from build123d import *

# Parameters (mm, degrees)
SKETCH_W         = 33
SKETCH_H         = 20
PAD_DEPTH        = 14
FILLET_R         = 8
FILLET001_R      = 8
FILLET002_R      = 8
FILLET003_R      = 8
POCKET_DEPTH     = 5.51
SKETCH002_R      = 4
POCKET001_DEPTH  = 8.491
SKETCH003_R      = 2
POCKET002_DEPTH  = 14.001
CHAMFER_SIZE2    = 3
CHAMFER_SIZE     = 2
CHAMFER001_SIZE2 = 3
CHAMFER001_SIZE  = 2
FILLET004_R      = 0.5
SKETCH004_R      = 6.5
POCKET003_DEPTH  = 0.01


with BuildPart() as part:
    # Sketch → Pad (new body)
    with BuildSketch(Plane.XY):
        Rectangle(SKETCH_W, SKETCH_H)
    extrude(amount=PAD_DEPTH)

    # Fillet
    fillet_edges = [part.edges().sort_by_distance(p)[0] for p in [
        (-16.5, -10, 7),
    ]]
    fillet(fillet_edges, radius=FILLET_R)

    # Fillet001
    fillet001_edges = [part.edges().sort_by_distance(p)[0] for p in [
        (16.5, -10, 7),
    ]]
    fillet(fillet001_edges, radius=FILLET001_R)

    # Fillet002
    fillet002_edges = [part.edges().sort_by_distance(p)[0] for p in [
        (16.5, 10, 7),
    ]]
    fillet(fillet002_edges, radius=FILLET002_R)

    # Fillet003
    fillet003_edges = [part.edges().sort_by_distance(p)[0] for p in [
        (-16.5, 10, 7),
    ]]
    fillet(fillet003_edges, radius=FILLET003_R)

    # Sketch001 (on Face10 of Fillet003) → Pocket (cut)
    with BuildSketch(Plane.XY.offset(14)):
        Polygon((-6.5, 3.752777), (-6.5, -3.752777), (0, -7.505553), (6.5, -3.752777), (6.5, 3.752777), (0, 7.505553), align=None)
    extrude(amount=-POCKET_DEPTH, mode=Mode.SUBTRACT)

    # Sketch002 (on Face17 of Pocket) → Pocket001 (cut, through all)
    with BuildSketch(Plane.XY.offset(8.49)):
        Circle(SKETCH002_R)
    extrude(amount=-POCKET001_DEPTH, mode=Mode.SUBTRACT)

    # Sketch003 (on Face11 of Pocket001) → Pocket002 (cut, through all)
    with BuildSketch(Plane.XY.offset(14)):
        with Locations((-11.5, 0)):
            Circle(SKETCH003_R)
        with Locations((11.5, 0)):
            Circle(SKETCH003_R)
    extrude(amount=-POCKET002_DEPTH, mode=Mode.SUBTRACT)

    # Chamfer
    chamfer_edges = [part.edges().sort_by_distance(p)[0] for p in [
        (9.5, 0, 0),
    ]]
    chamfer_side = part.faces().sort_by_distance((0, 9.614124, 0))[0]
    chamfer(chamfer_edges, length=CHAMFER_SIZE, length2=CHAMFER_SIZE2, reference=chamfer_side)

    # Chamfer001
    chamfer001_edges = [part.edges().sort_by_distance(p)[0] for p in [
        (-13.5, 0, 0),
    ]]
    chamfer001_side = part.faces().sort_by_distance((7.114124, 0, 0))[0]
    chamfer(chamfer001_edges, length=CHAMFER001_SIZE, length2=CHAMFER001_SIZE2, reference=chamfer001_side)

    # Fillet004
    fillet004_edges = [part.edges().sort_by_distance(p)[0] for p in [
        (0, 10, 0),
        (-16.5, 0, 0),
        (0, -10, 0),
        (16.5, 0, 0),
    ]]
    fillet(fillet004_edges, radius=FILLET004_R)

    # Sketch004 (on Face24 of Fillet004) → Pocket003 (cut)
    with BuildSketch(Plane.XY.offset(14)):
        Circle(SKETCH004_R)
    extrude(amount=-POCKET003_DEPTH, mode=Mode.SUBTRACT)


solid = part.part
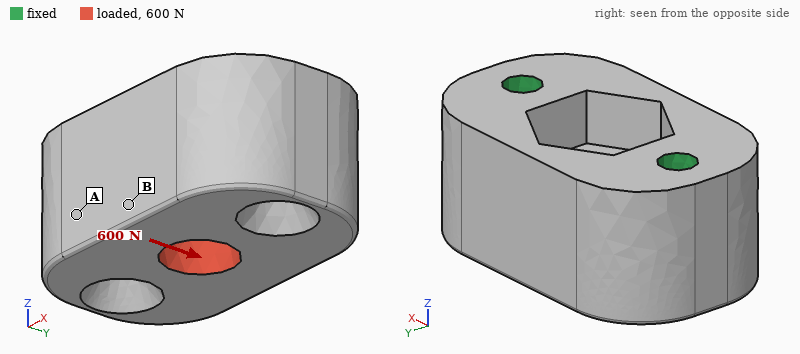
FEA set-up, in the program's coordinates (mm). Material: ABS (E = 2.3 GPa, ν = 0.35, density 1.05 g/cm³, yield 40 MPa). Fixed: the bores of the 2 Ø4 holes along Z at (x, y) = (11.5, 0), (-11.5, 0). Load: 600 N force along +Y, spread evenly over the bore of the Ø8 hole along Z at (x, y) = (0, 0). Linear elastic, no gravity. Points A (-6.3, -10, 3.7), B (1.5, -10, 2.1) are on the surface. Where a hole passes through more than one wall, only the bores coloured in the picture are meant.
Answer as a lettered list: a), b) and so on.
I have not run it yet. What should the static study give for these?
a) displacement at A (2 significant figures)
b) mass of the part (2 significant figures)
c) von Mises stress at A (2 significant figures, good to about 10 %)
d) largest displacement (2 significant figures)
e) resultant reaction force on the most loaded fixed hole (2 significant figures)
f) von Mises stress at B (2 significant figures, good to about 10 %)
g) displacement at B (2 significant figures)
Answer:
a) 23 µm
b) 7.1 g
c) 1.7 MPa
d) 38 µm
e) 300 N
f) 4.4 MPa
g) 32 µm
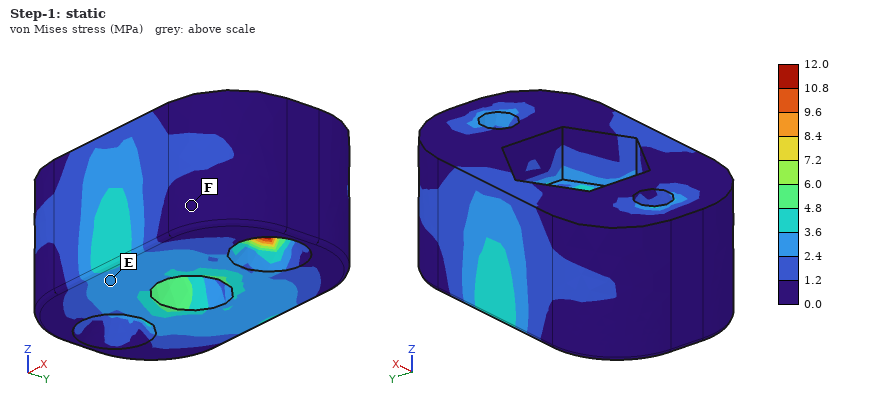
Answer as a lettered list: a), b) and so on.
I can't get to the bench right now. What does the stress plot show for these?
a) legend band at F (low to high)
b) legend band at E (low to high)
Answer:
a) 0.0 to 1.2 MPa
b) 2.4 to 3.6 MPa
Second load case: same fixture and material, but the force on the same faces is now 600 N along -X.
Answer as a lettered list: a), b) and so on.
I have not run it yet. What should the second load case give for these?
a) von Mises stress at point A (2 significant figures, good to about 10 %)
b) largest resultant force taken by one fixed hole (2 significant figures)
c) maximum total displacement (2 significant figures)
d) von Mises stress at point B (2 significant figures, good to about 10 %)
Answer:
a) 0.50 MPa
b) 300 N
c) 17 µm
d) 0.46 MPa
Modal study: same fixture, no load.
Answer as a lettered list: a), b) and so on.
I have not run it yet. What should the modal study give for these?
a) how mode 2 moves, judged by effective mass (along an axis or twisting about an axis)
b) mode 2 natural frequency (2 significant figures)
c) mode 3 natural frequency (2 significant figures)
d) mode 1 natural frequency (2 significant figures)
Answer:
a) along Z
b) 13 kHz
c) 16 kHz
d) 11 kHz
